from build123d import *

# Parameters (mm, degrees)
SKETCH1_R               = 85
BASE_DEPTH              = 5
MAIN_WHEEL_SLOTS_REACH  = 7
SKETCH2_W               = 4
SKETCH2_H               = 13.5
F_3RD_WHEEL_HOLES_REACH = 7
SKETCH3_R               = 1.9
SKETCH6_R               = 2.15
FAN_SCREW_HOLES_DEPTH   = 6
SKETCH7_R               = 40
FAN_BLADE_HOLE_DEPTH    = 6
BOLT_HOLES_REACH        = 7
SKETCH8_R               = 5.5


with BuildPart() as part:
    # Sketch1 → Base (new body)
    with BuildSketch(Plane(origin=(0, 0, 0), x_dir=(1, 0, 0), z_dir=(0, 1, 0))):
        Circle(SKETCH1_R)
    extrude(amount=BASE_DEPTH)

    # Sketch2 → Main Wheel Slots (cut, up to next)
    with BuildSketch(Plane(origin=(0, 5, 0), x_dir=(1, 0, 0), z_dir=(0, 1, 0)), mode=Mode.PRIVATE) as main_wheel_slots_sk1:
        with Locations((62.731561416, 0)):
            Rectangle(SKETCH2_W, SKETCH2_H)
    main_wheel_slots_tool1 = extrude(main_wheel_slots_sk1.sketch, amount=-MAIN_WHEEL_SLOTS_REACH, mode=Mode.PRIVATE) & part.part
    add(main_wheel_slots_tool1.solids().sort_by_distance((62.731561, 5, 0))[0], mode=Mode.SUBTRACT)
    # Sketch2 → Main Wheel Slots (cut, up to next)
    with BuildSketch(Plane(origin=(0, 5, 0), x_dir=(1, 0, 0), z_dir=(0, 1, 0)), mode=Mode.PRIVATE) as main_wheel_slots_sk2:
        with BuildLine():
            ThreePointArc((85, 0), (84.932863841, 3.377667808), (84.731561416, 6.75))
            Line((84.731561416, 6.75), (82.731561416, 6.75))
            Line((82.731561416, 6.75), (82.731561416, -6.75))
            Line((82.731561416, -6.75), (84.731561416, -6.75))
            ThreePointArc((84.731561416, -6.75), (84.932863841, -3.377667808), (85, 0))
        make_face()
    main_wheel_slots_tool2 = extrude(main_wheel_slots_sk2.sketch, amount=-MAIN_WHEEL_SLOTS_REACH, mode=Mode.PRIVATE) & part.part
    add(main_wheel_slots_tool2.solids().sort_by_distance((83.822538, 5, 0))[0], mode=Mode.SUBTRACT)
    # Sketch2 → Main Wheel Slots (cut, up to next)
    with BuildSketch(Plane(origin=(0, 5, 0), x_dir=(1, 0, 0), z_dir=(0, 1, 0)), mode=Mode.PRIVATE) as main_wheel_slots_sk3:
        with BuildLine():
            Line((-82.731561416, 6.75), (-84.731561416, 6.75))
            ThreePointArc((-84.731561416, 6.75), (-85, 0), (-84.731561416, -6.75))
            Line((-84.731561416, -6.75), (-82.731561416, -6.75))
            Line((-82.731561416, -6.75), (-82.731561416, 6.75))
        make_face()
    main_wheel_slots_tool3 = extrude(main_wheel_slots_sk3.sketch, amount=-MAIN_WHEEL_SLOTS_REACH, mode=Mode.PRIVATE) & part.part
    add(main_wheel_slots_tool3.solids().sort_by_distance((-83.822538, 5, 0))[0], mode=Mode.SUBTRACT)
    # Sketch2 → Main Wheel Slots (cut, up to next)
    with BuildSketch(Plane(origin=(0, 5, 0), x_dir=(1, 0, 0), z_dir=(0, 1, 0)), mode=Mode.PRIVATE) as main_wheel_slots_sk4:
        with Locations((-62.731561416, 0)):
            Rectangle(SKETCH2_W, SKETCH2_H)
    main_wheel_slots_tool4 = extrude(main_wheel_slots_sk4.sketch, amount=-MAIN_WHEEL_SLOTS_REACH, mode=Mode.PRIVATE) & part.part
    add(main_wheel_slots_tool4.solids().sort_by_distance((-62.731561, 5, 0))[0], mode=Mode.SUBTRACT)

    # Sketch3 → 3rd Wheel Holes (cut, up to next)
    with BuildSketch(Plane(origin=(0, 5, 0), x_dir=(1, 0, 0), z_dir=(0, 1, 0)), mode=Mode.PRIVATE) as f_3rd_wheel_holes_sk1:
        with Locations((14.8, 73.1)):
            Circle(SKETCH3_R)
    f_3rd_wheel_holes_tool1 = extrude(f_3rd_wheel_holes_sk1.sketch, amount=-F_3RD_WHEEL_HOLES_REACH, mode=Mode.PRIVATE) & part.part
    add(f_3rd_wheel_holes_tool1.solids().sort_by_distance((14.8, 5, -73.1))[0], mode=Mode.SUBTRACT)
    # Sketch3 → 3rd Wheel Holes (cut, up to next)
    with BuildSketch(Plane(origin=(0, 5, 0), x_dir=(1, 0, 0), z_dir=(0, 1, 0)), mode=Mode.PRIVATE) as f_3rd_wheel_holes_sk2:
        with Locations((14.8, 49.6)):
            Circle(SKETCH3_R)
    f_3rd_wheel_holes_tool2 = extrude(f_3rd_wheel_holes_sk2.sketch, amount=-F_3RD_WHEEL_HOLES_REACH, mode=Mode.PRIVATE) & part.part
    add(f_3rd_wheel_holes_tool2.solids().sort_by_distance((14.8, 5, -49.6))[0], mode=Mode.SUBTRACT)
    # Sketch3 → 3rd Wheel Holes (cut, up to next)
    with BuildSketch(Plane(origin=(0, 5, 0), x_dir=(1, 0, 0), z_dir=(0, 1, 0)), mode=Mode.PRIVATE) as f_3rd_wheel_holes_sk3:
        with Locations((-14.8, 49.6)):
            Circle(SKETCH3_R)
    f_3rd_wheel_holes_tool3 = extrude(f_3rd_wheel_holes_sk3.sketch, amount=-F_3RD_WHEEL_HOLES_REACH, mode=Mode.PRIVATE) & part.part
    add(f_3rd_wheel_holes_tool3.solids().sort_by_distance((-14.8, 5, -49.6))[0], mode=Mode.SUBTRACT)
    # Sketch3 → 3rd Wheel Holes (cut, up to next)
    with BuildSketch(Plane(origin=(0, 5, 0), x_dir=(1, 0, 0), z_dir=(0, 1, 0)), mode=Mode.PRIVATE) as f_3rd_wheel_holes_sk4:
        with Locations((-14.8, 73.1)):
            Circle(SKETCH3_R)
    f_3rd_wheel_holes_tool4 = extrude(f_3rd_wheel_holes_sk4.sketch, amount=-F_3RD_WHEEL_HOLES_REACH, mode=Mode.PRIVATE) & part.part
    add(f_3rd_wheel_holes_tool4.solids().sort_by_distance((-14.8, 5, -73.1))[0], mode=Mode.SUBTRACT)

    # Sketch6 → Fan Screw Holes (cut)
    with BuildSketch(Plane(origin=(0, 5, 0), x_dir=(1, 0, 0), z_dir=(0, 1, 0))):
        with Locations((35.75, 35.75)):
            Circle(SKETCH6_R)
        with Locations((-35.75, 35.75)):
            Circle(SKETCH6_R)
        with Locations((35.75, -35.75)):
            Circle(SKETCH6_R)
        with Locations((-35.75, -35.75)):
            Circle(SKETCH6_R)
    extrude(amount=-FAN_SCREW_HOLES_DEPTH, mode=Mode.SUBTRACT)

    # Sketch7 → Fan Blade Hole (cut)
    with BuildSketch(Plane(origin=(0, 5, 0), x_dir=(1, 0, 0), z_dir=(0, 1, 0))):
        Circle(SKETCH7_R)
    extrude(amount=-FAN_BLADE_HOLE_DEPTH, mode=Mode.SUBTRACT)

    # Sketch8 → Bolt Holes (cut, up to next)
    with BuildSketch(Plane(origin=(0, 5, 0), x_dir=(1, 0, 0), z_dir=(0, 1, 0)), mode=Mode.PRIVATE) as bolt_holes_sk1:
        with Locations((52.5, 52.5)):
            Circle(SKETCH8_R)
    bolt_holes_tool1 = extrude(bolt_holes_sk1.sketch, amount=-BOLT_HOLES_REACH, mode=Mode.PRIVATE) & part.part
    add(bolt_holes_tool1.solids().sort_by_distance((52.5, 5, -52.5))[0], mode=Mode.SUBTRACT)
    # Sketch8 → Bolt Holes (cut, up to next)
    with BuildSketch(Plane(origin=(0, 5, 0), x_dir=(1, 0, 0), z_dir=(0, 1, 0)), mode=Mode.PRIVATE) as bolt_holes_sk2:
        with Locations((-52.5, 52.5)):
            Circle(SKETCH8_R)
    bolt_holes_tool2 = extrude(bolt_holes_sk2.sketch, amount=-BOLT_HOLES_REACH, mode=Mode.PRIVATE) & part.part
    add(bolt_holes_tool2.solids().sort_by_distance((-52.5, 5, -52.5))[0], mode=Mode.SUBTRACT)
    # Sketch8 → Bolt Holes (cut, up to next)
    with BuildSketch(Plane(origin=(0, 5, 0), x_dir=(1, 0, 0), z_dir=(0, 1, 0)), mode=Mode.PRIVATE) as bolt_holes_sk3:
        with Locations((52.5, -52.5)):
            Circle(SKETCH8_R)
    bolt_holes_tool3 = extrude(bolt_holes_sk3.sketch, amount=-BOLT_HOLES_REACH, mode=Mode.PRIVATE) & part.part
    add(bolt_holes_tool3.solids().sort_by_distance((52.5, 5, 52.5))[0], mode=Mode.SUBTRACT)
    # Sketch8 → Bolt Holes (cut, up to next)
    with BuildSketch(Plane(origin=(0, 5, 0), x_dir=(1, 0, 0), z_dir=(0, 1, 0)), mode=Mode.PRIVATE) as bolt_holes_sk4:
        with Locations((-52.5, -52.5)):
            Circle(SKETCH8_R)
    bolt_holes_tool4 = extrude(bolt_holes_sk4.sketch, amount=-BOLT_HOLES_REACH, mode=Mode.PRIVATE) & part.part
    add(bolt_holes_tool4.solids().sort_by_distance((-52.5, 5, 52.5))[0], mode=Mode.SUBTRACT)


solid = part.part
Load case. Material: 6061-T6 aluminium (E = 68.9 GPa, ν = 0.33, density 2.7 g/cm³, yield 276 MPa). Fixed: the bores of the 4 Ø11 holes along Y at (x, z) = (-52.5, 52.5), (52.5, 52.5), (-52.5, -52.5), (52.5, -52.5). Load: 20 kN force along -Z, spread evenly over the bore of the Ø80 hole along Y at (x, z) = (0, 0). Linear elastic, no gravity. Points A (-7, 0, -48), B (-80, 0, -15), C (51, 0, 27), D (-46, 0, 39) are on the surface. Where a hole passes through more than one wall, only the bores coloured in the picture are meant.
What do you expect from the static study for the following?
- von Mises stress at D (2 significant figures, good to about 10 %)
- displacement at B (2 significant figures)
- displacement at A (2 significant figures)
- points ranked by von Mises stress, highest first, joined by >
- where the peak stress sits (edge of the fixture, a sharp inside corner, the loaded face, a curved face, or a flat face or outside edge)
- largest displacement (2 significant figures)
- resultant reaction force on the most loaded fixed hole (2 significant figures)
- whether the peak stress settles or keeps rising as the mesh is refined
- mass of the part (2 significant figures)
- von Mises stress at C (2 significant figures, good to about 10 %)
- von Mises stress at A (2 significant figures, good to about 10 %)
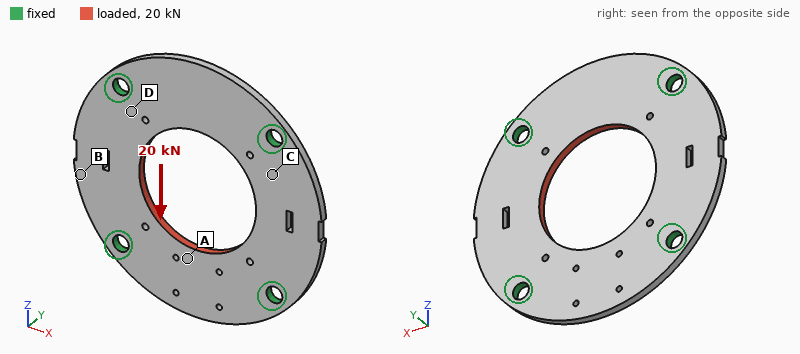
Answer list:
33 MPa
5.6 µm
30 µm
D > C > A > B
edge of the fixture
32 µm
5.0 kN
keeps rising
230 g
22 MPa
15 MPa
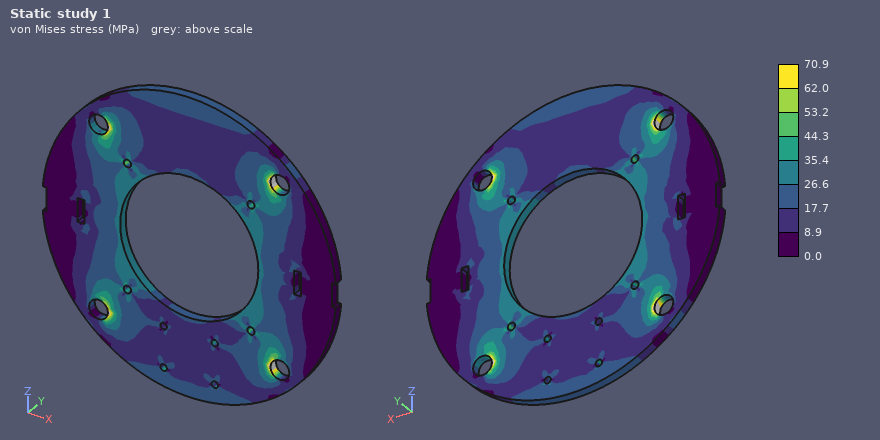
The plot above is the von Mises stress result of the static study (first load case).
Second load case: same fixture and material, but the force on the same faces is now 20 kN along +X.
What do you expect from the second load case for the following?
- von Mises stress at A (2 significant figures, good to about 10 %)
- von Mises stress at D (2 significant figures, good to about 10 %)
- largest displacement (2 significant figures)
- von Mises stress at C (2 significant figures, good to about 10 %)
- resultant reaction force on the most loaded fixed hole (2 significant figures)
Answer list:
23 MPa
26 MPa
33 µm
18 MPa
5.0 kN
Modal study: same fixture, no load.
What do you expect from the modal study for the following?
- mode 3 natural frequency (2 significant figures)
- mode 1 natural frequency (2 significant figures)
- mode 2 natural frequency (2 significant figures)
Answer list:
2200 Hz
2100 Hz
2200 Hz
